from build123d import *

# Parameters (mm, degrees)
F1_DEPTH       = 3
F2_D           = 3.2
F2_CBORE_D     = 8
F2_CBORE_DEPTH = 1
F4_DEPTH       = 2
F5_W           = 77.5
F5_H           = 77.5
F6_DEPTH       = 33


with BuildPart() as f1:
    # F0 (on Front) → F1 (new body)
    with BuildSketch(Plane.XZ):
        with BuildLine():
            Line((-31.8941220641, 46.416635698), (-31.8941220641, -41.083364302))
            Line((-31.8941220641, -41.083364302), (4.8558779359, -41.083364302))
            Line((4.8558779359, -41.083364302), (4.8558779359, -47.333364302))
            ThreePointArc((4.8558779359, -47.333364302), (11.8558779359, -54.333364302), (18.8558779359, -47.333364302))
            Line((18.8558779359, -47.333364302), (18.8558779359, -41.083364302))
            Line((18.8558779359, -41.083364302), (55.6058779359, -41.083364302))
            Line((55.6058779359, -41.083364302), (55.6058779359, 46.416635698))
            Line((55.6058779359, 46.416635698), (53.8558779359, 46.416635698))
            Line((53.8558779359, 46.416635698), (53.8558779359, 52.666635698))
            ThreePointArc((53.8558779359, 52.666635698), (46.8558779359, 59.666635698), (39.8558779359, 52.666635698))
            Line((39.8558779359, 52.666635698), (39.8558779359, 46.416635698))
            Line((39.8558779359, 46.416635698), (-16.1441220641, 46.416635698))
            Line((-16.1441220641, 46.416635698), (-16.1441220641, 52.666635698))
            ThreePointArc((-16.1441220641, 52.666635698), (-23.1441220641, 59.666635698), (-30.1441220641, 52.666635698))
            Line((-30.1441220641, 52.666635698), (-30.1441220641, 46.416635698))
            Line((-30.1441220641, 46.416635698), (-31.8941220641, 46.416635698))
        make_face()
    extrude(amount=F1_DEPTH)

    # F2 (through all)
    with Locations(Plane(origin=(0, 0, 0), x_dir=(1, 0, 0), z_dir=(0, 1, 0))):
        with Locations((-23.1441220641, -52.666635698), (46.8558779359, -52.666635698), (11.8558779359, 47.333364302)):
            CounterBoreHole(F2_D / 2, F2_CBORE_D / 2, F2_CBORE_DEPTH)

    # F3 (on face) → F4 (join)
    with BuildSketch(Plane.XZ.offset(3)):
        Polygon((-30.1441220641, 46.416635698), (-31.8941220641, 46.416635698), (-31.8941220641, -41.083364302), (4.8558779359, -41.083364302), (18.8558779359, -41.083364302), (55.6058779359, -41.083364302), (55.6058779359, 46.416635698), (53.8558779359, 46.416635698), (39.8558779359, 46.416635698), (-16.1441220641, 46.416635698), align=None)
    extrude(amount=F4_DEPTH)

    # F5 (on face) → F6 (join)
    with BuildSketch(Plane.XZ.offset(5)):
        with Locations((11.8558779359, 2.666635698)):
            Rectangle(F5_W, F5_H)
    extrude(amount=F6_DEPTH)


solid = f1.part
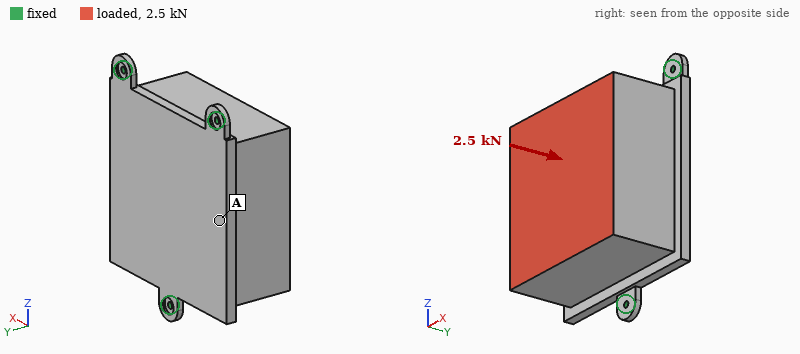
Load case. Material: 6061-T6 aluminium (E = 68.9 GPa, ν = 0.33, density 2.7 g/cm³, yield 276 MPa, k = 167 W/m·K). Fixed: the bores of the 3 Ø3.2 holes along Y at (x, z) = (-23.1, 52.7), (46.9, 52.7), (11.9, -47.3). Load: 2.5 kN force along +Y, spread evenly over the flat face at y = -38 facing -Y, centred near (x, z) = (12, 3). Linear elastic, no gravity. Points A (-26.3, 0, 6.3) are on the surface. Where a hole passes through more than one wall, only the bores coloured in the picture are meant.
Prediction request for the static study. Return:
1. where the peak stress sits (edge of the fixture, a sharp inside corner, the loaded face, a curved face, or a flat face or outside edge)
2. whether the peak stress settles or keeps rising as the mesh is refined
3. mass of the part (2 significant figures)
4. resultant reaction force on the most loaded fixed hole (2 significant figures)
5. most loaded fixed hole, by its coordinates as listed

edge of the fixture
keeps rising
640 g
1.4 kN
(11.9, -47.3)
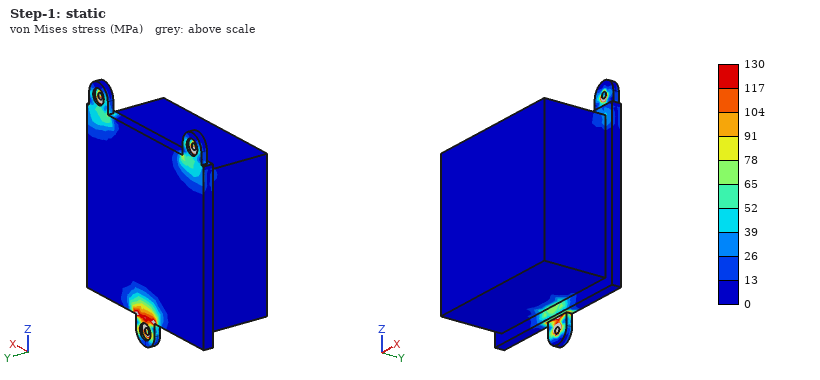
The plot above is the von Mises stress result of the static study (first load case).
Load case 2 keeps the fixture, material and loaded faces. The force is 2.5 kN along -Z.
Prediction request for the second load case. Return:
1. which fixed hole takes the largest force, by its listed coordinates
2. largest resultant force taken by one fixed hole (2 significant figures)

(11.9, -47.3)
1.4 kN
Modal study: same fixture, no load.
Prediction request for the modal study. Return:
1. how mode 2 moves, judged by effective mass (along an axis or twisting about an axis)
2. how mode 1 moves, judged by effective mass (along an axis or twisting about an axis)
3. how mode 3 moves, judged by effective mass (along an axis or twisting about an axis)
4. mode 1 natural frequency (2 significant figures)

along Y
along X
along Z
1200 Hz
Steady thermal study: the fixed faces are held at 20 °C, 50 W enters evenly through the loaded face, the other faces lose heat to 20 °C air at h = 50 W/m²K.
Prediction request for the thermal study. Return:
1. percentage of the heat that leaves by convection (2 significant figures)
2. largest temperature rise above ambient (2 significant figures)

41 %
21 K
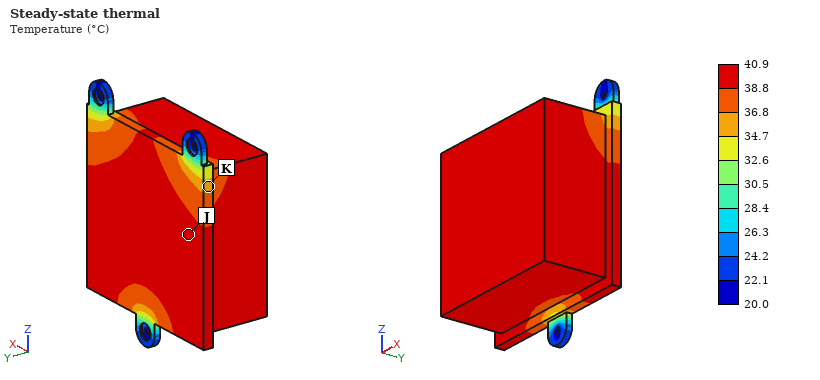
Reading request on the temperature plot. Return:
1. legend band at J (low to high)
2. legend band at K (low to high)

38.8 to 40.9 °C
34.7 to 36.8 °C
